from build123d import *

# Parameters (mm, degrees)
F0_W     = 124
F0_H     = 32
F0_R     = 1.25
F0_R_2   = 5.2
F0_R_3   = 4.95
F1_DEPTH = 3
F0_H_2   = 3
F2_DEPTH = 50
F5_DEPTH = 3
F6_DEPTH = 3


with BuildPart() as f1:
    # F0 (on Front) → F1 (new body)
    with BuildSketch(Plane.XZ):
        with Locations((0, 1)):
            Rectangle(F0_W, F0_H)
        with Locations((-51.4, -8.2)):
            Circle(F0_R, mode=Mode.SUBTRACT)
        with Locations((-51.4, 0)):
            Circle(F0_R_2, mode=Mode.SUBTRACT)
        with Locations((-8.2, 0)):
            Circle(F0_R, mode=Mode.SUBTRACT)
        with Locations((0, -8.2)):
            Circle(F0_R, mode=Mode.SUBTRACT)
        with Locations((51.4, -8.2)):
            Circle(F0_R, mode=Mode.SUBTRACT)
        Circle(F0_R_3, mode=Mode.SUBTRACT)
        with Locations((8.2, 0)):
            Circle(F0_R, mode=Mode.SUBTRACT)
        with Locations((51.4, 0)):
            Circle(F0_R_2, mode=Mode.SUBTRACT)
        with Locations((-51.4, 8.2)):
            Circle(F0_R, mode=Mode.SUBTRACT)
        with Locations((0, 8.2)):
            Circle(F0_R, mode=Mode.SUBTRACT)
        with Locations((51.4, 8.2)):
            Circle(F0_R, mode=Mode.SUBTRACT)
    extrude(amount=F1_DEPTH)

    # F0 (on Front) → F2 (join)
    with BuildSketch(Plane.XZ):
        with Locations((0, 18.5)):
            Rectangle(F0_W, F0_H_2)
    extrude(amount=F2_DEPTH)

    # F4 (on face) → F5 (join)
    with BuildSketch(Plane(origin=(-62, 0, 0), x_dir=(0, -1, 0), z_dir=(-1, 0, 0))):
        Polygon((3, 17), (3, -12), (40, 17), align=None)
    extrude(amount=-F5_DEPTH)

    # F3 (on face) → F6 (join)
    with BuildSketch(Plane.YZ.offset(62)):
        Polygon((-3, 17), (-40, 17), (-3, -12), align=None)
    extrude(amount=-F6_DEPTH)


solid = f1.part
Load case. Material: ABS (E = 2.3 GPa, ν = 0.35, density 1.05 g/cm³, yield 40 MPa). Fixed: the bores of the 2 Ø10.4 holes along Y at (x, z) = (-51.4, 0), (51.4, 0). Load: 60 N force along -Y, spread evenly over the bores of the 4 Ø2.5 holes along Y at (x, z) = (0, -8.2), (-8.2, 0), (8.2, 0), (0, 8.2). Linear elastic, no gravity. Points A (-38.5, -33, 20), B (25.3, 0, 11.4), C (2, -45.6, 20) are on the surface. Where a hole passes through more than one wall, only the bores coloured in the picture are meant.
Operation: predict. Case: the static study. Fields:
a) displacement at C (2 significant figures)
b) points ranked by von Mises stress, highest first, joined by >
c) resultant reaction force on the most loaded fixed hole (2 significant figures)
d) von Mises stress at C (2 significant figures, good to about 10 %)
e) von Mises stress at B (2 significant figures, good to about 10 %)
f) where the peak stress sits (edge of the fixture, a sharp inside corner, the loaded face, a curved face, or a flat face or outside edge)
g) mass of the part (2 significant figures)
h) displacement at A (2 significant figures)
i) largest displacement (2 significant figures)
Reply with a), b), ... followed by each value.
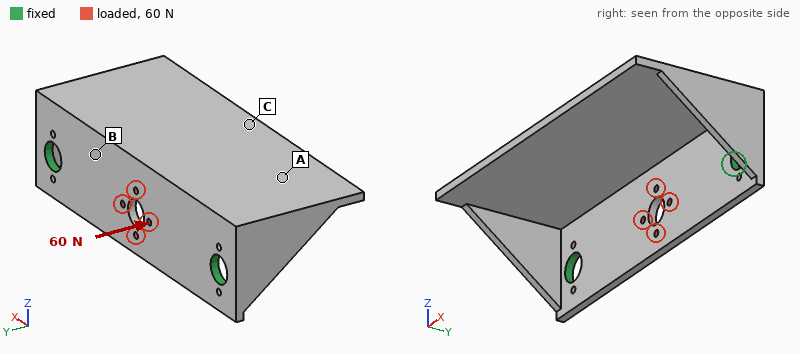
a) 0.47 mm
b) B > C > A
c) 31 N
d) 1.9 MPa
e) 4.3 MPa
f) the loaded face
g) 35 g
h) 0.17 mm
i) 1.0 mm
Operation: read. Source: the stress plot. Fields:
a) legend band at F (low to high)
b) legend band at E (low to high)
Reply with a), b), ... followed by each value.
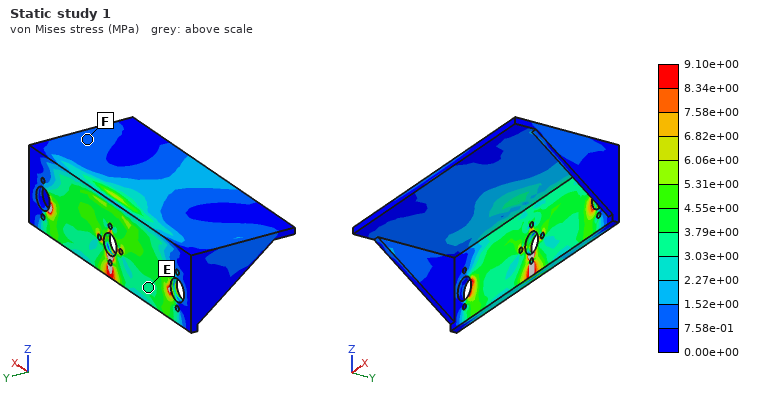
a) 7.58e-01 to 1.52e+00 MPa
b) 3.03e+00 to 3.79e+00 MPa
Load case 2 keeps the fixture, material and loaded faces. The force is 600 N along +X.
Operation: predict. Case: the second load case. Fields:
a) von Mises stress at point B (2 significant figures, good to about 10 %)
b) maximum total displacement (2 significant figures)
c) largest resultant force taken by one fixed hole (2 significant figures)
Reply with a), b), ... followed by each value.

a) 2.2 MPa
b) 83 µm
c) 300 N
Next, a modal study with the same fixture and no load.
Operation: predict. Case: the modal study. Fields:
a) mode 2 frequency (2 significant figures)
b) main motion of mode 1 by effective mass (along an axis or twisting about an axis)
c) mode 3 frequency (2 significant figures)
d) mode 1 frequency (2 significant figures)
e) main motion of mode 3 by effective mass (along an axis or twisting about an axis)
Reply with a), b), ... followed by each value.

a) 560 Hz
b) along Z
c) 710 Hz
d) 300 Hz
e) along Y
